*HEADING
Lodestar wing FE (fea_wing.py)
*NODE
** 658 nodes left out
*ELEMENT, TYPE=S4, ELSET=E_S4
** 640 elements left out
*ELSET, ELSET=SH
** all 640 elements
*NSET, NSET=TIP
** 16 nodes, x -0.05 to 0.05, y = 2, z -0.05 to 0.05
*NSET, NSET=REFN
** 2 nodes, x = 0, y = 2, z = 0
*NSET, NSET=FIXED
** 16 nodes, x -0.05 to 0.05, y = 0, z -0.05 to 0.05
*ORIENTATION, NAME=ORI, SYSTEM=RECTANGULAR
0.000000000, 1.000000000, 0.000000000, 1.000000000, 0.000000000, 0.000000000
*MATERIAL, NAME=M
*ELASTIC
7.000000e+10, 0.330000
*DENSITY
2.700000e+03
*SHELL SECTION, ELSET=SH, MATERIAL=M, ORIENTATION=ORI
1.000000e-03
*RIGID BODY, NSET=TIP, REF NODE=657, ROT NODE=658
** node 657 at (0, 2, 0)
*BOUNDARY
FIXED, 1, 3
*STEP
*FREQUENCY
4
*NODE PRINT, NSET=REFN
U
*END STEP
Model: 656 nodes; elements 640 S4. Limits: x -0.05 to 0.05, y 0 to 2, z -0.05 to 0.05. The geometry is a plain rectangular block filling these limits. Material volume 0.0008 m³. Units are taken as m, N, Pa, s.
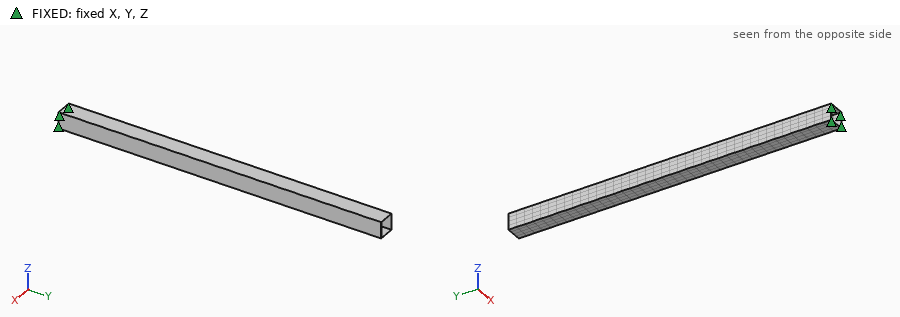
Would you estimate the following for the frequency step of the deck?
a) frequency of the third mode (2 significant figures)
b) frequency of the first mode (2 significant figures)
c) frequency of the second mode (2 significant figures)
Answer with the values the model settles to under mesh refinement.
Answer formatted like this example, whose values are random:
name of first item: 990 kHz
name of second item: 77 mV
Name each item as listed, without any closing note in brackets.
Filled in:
frequency of the third mode: 170 Hz
frequency of the first mode: 29 Hz
frequency of the second mode: 29 Hz
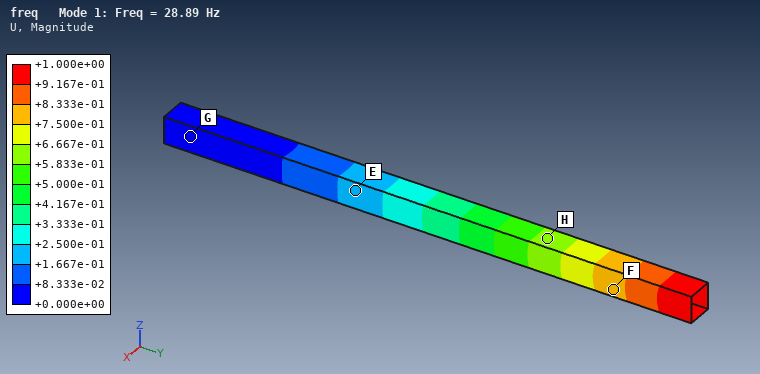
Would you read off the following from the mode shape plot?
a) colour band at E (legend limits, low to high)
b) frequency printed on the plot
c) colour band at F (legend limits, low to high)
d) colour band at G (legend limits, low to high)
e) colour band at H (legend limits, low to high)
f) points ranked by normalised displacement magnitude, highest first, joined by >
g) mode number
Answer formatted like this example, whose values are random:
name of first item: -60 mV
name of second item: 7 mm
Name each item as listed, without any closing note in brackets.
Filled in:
colour band at E: +1.667e-01 to +2.500e-01
frequency printed on the plot: 28.89 Hz
colour band at F: +7.500e-01 to +8.333e-01
colour band at G: +0.000e+00 to +8.333e-02
colour band at H: +5.833e-01 to +6.667e-01
points ranked by normalised displacement magnitude, highest first, joined by >: F > H > E > G
mode number: 1
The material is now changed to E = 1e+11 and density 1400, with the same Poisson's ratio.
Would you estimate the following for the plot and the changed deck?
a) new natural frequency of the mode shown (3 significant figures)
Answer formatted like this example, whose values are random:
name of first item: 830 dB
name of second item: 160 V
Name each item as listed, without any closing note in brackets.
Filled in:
new natural frequency of the mode shown: 48.0 Hz
